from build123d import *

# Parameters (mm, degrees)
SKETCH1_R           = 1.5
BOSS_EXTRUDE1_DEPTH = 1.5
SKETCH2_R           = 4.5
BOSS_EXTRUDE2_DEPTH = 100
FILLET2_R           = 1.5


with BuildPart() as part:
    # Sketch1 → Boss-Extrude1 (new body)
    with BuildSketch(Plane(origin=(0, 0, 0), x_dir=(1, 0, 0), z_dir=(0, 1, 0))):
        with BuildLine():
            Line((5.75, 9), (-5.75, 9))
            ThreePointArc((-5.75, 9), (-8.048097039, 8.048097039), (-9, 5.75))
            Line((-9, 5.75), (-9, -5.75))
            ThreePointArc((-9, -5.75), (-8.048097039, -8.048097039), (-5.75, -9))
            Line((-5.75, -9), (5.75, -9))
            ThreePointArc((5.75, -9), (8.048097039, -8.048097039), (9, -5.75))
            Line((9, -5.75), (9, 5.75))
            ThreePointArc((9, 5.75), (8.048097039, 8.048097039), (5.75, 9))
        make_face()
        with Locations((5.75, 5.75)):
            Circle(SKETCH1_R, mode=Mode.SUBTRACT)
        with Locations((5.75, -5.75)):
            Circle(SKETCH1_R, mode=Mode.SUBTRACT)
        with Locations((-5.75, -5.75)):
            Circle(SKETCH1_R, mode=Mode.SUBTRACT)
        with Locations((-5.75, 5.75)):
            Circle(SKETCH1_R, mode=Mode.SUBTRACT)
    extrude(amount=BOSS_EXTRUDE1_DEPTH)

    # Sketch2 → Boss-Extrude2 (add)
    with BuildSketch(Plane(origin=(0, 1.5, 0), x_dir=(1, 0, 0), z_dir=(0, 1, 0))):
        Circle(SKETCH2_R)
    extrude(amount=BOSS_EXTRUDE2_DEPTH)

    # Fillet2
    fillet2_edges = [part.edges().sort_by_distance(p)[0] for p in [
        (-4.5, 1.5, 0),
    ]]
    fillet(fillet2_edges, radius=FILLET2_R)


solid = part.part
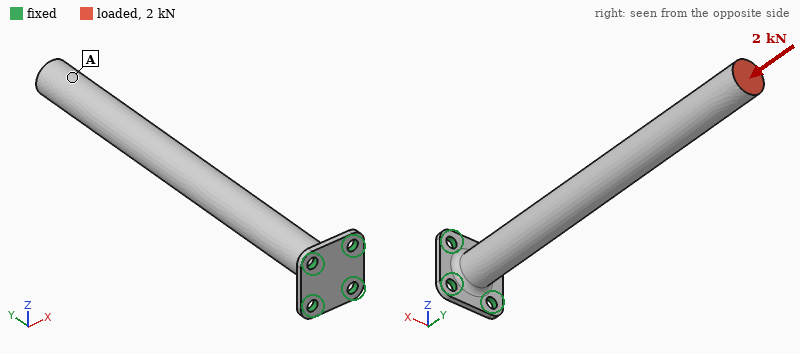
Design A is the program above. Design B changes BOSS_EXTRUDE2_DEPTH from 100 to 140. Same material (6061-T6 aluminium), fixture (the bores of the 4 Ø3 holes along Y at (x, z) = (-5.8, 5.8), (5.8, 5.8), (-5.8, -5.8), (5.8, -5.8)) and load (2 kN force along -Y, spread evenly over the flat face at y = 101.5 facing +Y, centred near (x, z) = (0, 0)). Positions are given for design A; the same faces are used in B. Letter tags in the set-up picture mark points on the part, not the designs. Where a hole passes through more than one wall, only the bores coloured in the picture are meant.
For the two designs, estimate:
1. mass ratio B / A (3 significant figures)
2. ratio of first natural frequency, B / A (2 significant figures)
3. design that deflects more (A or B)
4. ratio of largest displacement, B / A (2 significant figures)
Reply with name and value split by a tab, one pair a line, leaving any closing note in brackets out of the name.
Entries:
mass ratio B / A	1.37
ratio of first natural frequency, B / A	0.53
design that deflects more	B
ratio of largest displacement, B / A	1.3
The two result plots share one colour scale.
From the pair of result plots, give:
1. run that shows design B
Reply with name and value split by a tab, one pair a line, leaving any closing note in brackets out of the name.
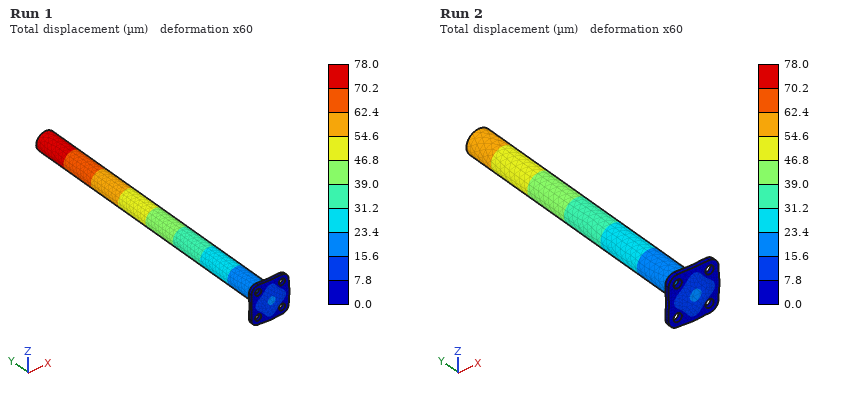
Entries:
run that shows design B	Run 1
